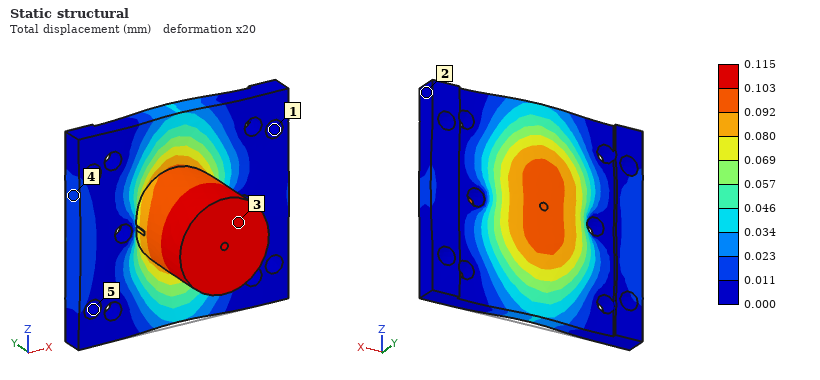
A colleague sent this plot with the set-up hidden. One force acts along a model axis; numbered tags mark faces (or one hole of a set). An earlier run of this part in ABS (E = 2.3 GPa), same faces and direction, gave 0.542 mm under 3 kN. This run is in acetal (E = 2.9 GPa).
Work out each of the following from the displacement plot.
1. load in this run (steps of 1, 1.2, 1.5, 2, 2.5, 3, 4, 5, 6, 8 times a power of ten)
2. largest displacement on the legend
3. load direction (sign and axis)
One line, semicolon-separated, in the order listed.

800 N; 0.115 mm; +Y
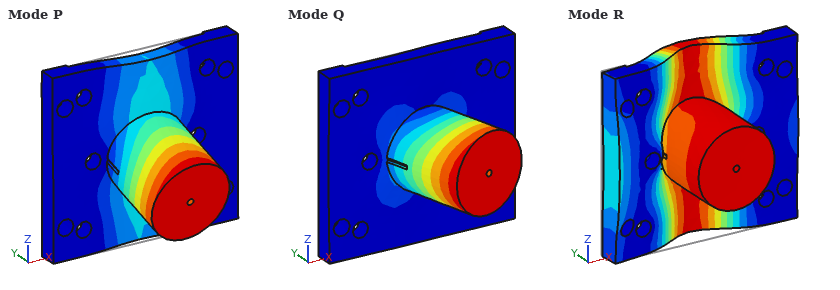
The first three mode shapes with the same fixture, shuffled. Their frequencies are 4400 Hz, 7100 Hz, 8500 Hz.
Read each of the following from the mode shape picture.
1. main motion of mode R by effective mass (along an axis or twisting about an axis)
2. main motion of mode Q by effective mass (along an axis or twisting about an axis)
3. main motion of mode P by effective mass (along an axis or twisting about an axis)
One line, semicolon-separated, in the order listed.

along Y; along X; along Z
